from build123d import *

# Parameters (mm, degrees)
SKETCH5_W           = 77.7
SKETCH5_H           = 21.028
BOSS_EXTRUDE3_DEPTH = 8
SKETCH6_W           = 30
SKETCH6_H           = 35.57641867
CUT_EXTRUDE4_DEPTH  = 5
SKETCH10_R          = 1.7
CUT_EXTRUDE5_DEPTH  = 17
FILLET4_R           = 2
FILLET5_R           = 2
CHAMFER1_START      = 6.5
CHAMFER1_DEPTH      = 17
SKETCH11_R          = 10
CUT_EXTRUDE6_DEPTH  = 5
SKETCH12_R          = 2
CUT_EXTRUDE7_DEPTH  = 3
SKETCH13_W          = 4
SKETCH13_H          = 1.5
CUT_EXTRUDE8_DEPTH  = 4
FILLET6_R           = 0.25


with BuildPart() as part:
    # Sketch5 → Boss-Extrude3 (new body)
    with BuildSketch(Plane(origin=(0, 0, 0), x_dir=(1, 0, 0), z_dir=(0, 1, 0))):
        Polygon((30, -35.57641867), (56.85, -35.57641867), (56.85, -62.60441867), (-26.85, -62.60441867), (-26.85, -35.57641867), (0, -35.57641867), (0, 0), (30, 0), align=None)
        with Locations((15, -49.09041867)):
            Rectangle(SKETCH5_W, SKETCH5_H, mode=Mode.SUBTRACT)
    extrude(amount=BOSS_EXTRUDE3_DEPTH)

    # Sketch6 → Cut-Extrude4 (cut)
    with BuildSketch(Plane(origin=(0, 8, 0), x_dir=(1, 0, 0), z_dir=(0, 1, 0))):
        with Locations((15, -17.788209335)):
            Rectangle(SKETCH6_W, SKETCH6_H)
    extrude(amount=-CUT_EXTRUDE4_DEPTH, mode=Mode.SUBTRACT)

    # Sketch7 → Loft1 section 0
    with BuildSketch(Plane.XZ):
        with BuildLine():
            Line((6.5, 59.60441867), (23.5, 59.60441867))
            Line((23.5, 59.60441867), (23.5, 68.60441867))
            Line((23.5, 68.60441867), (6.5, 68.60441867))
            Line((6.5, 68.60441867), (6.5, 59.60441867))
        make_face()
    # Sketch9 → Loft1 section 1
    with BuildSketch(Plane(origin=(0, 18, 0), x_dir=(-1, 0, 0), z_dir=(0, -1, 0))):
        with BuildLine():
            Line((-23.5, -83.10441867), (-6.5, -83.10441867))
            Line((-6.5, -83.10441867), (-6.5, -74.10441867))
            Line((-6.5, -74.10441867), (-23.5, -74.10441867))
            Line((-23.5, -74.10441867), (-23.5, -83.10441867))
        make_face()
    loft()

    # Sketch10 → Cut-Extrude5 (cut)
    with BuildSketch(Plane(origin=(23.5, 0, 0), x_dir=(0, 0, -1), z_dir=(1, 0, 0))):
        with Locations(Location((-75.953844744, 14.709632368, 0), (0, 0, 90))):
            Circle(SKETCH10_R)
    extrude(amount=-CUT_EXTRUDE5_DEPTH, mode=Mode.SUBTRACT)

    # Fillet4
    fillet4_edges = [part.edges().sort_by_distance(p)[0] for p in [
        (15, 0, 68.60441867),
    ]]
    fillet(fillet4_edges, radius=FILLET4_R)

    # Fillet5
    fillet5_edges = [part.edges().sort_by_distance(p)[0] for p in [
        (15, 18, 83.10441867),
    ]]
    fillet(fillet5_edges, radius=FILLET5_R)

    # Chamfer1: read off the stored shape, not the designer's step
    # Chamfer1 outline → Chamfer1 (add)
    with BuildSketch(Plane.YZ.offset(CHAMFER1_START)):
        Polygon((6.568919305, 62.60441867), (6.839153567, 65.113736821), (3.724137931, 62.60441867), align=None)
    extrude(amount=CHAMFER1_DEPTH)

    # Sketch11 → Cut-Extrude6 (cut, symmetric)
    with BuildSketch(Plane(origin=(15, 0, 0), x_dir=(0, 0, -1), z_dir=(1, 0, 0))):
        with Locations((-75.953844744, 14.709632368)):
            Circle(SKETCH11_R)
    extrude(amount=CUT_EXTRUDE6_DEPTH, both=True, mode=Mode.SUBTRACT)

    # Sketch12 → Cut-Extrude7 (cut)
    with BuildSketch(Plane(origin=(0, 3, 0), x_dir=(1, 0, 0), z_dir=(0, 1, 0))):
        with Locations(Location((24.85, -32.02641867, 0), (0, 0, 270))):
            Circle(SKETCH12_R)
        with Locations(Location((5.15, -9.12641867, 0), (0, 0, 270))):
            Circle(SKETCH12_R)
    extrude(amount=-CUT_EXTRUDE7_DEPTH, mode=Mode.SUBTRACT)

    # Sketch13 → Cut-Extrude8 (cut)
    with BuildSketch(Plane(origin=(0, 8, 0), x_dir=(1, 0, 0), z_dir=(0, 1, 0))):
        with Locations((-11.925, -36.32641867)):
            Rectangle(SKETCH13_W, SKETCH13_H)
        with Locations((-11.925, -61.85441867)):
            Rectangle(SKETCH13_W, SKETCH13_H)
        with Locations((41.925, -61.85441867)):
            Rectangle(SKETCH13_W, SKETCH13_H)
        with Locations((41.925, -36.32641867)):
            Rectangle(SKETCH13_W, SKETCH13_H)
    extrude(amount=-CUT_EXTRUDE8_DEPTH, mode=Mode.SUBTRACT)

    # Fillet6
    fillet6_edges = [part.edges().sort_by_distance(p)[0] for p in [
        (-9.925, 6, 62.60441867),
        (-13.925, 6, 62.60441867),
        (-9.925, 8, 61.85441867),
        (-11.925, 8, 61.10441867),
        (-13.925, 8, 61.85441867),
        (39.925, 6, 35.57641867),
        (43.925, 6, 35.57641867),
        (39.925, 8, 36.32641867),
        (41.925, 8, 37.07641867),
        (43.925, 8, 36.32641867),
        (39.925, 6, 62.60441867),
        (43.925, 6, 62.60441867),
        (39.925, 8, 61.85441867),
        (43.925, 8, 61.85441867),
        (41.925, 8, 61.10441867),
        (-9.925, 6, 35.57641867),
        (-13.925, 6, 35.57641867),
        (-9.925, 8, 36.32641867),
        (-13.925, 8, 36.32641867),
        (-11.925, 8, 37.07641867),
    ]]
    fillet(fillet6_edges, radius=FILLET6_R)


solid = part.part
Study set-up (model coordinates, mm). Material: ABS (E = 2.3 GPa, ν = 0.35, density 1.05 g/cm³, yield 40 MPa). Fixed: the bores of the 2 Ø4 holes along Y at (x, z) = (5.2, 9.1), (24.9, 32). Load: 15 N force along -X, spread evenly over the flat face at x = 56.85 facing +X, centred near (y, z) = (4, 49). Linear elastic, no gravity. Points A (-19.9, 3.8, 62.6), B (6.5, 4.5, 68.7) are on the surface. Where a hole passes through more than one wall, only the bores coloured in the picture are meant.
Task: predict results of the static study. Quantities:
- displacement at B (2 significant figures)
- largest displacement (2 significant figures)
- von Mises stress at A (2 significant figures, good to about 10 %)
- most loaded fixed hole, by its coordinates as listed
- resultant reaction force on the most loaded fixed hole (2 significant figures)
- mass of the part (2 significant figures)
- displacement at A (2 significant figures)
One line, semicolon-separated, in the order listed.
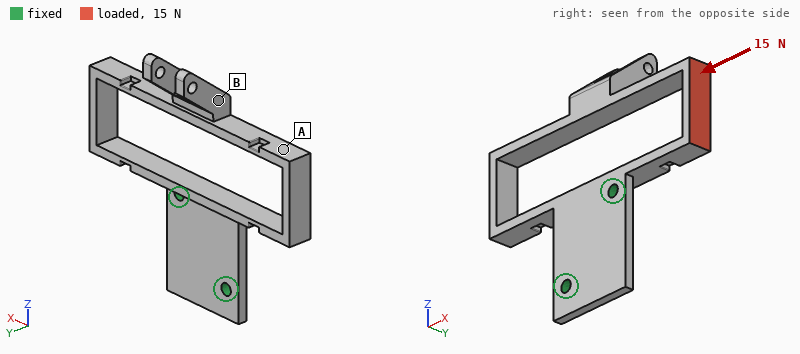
1.1 mm; 1.4 mm; 3.5 MPa; (24.9, 32); 19 N; 10 g; 1.2 mm
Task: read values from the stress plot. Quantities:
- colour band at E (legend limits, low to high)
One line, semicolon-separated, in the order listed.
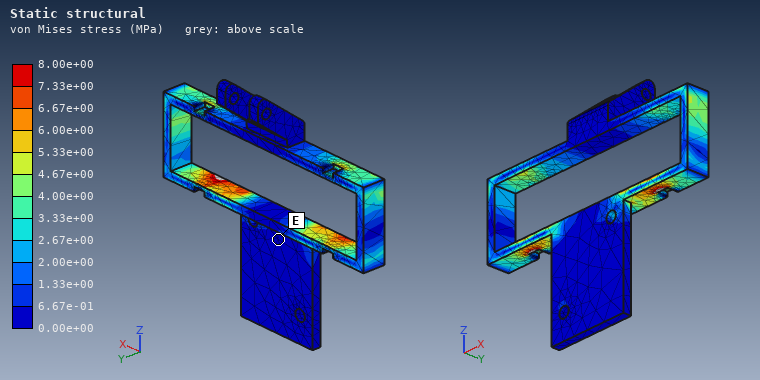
0.00e+00 to 6.67e-01 MPa
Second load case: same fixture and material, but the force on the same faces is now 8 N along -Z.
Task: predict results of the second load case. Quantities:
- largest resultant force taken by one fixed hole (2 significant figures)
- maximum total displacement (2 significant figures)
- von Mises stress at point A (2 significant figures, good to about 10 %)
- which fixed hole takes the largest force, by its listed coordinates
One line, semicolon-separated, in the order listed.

15 N; 1.4 mm; 1.9 MPa; (24.9, 32)
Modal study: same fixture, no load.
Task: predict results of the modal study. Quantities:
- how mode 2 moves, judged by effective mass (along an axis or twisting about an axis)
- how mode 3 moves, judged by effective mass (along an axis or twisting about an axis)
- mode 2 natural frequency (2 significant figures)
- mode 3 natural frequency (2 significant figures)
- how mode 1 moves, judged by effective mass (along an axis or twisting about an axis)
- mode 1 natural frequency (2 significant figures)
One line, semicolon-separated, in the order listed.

along X; along Z; 190 Hz; 260 Hz; along Y; 130 Hz
